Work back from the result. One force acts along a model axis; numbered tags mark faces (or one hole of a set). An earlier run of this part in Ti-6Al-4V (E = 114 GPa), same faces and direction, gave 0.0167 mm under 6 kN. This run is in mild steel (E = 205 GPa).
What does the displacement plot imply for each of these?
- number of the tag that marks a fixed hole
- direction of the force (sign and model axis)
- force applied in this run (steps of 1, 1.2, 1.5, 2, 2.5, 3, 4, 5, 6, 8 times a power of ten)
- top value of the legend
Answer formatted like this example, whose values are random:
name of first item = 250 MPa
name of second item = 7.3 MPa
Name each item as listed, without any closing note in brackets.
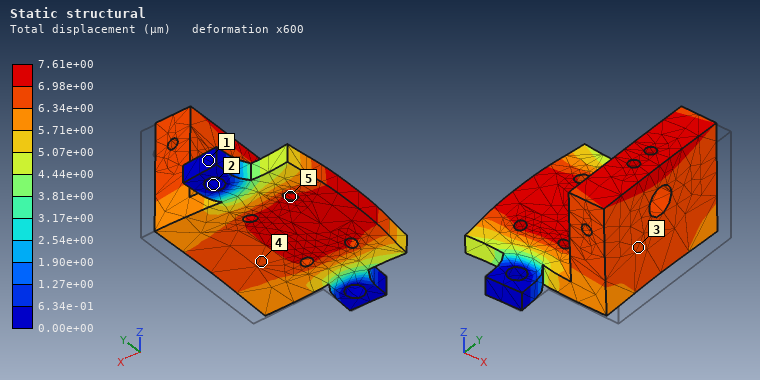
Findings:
number of the tag that marks a fixed hole = 2
direction of the force = -X
force applied in this run = 5 kN
top value of the legend = 7.61e+00 µm
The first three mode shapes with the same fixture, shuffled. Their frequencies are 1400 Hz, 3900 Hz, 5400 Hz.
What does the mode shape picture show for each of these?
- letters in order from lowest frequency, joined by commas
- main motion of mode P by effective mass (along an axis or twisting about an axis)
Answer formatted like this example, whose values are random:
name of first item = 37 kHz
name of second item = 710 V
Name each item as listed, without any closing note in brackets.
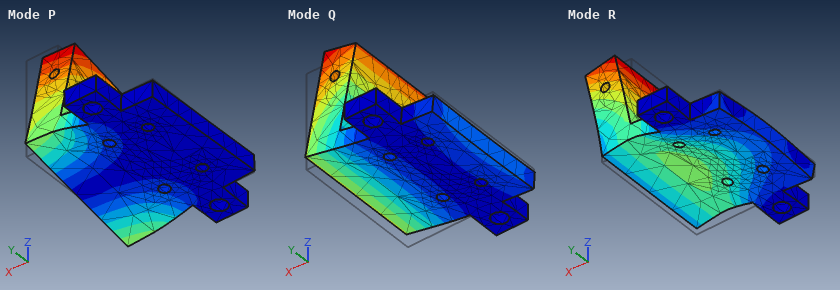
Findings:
letters in order from lowest frequency, joined by commas = Q, P, R
main motion of mode P by effective mass = along Y
